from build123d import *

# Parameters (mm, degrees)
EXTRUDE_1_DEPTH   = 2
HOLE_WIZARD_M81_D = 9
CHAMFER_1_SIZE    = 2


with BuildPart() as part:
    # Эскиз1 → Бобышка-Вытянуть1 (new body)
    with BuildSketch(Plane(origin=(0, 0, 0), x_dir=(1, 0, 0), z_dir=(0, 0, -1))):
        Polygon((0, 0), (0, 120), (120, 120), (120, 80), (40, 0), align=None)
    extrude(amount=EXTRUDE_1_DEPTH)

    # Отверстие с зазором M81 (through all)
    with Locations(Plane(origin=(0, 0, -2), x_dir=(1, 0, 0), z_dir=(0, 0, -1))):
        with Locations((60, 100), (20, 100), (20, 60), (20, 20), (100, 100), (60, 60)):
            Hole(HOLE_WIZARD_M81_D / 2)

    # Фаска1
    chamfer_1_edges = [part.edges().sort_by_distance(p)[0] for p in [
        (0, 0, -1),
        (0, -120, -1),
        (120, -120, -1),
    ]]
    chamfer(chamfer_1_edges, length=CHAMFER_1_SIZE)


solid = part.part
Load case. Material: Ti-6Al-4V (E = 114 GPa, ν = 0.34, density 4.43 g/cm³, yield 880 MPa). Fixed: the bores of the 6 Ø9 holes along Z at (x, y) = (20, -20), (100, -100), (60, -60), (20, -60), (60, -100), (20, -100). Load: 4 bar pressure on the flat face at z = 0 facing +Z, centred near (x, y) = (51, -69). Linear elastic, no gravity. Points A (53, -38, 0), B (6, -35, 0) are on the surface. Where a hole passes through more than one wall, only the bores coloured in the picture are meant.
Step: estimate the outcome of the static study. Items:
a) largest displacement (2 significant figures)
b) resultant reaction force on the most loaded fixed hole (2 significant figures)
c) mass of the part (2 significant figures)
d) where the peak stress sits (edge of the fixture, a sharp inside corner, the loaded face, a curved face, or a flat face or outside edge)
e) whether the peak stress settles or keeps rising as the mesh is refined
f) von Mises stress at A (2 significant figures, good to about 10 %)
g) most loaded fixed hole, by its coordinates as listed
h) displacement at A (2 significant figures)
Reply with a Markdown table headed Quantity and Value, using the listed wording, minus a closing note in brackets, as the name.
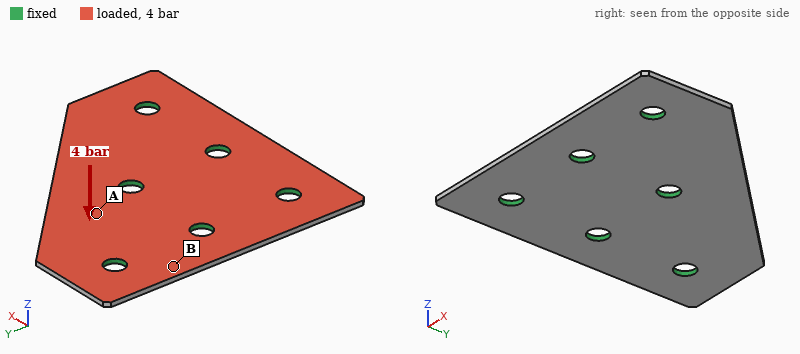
| Quantity | Value |
|---|---|
| largest displacement | 0.44 mm |
| resultant reaction force on the most loaded fixed hole | 1.0 kN |
| mass of the part | 96 g |
| where the peak stress sits | edge of the fixture |
| whether the peak stress settles or keeps rising as the mesh is refined | keeps rising |
| von Mises stress at A | 76 MPa |
| most loaded fixed hole, by its coordinates as listed | (60, -60) |
| displacement at A | 0.16 mm |
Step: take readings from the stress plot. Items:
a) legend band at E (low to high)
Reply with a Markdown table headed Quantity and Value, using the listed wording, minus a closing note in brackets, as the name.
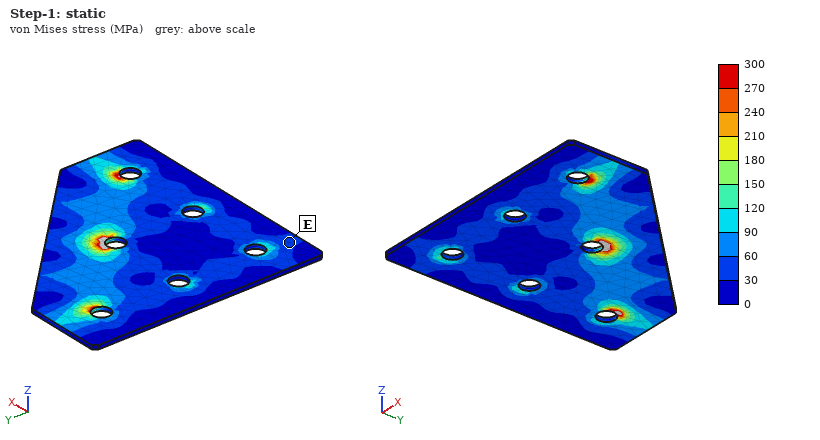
| Quantity | Value |
|---|---|
| legend band at E | 30 to 60 MPa |
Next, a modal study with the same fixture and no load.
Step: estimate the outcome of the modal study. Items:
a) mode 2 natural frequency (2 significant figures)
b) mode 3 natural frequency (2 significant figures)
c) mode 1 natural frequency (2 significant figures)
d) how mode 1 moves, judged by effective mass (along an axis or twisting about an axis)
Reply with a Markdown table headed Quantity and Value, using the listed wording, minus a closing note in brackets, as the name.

| Quantity | Value |
|---|---|
| mode 2 natural frequency | 2400 Hz |
| mode 3 natural frequency | 3900 Hz |
| mode 1 natural frequency | 2100 Hz |
| how mode 1 moves, judged by effective mass | along Z |
